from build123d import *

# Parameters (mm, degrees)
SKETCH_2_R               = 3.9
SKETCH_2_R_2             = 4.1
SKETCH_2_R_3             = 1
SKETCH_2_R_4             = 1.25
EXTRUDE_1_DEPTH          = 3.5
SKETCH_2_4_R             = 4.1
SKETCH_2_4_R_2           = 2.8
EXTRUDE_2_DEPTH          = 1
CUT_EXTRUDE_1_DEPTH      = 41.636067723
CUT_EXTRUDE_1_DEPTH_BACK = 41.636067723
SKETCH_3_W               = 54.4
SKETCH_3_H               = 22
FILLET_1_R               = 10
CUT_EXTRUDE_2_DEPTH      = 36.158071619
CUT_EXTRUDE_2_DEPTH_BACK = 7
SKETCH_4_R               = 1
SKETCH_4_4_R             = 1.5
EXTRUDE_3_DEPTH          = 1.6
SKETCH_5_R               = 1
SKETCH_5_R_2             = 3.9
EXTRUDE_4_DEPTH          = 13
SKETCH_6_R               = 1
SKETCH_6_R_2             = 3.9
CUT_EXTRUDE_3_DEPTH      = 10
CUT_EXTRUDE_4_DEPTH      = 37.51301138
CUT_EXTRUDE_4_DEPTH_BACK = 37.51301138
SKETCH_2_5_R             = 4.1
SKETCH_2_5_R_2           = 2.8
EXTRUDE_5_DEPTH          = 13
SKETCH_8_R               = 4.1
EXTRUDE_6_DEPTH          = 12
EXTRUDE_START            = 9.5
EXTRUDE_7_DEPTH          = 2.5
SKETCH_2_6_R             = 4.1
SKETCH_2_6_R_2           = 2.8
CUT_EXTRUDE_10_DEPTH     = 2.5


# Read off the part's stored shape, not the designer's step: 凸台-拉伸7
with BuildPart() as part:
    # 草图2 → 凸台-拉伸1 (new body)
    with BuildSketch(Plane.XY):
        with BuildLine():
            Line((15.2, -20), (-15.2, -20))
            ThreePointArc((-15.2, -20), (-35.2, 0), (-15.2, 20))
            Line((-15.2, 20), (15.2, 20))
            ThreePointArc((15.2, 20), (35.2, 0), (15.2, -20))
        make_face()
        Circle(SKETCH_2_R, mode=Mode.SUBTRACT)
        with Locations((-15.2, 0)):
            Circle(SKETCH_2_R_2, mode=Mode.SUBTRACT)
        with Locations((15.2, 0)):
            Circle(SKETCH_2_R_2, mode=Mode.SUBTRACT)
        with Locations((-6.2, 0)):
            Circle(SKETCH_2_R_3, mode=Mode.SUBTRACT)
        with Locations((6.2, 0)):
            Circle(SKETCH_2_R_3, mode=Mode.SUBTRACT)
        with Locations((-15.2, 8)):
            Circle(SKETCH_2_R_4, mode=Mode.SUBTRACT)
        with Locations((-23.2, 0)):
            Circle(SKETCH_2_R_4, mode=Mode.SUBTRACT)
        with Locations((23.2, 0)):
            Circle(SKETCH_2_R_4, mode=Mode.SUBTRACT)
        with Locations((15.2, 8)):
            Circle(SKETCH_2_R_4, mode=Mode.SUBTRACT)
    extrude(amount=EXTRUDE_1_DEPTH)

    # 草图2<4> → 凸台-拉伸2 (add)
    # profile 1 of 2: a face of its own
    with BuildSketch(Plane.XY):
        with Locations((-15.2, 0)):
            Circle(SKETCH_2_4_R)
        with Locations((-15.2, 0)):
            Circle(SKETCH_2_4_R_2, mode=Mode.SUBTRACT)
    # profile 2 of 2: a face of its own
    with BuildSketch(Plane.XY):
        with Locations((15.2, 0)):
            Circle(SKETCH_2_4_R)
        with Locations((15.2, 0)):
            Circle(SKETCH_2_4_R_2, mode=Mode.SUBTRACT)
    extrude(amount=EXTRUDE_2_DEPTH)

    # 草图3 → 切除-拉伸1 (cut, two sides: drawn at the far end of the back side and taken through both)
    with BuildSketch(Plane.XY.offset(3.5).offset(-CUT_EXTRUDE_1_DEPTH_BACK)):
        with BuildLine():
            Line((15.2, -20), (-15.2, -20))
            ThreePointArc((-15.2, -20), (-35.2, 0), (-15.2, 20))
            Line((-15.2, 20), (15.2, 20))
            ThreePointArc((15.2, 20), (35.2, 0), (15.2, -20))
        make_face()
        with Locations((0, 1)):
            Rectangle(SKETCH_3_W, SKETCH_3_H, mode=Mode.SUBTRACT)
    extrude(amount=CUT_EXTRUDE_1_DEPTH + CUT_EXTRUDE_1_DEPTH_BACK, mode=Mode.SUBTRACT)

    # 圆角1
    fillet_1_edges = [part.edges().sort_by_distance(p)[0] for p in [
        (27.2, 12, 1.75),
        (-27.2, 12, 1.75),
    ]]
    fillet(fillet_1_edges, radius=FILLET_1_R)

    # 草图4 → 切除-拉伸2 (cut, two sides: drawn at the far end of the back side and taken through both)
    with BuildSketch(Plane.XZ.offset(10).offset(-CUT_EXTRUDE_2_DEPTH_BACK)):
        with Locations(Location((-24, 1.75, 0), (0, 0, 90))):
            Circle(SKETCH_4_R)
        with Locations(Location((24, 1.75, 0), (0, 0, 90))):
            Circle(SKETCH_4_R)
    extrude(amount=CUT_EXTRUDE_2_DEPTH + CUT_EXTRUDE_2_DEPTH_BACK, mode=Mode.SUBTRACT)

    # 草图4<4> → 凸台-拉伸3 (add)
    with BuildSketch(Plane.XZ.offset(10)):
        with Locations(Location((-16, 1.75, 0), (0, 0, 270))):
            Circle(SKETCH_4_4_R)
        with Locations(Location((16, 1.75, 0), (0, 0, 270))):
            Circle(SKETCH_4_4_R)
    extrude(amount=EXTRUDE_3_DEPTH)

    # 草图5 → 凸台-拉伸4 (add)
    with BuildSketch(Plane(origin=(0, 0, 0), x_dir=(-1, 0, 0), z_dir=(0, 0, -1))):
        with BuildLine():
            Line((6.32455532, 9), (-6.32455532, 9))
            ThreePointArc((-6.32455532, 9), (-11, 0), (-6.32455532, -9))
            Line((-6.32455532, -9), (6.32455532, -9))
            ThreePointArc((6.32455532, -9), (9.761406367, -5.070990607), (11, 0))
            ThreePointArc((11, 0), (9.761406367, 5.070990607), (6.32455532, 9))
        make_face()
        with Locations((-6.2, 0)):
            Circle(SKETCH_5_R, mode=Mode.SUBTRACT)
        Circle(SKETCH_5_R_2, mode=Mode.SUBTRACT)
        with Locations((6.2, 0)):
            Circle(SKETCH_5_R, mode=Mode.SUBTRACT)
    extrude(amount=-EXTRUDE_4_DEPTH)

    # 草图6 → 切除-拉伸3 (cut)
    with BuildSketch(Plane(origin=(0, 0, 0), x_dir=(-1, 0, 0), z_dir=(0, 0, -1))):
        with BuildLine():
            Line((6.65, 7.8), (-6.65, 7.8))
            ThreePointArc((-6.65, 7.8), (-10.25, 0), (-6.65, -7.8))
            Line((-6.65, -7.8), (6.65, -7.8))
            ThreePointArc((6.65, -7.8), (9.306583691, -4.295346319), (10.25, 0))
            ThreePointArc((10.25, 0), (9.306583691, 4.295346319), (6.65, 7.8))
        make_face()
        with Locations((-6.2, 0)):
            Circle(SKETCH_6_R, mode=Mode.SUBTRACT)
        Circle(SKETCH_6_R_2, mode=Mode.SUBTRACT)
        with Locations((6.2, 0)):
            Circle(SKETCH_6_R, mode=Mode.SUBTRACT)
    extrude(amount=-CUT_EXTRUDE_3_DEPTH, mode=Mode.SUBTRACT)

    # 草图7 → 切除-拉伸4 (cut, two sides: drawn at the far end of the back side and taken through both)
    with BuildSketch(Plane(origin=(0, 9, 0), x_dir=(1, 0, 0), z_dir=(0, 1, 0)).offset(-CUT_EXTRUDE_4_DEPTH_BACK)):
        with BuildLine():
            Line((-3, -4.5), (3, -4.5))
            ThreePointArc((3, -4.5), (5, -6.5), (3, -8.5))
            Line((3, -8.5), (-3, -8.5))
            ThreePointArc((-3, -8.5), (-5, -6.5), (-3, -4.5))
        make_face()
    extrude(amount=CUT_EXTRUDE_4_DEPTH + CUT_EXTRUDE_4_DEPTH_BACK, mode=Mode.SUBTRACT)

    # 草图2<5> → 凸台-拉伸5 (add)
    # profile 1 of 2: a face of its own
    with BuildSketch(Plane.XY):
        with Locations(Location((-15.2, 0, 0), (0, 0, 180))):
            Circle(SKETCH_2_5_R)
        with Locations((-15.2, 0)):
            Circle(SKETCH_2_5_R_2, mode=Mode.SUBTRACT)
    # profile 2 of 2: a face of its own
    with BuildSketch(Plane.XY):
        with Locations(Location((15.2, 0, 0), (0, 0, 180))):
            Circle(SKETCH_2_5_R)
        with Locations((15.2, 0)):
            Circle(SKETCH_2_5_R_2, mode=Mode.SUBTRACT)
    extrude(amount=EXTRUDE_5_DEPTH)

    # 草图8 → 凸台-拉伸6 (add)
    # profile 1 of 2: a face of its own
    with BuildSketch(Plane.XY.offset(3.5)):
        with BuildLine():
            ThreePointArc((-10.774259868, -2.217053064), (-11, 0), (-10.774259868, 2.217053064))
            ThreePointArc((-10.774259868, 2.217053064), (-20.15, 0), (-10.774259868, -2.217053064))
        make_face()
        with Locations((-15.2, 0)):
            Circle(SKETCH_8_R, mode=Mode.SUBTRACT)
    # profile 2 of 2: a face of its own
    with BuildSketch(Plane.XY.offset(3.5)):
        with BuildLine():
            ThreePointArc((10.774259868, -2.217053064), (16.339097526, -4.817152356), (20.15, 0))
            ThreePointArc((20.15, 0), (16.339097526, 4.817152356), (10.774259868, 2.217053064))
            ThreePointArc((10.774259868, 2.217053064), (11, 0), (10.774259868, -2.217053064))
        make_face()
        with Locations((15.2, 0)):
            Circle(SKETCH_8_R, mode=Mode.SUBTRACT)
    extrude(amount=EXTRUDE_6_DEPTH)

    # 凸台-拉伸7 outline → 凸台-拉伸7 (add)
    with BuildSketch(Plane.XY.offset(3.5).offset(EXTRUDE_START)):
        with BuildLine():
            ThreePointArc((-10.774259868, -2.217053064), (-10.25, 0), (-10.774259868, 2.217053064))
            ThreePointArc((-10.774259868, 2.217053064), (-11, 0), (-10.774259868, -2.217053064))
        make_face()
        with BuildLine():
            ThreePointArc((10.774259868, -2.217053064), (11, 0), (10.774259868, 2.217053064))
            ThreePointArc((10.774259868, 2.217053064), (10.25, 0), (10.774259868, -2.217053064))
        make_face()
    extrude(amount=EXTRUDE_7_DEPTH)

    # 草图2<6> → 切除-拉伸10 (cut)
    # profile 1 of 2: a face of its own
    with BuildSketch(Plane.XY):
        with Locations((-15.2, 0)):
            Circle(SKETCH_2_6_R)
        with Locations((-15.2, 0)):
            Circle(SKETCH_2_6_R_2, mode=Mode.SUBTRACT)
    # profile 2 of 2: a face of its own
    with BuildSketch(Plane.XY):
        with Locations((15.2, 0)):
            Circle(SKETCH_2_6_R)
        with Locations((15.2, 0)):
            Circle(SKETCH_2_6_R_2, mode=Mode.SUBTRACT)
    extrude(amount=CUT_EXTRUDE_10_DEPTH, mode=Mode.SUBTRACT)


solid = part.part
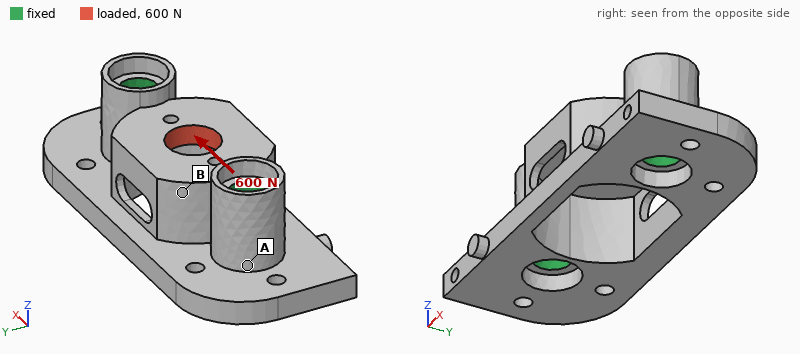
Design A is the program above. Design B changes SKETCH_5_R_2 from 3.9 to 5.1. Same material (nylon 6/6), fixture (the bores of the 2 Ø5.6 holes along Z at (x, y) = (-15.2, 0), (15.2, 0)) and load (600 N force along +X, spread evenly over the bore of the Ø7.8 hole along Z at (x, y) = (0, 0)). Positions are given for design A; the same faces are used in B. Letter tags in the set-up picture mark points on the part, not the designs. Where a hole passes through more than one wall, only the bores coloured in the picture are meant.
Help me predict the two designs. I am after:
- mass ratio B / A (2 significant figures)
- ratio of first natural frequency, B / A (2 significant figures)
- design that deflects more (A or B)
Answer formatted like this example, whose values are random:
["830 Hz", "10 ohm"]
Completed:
["0.98", "1.0", "B"]
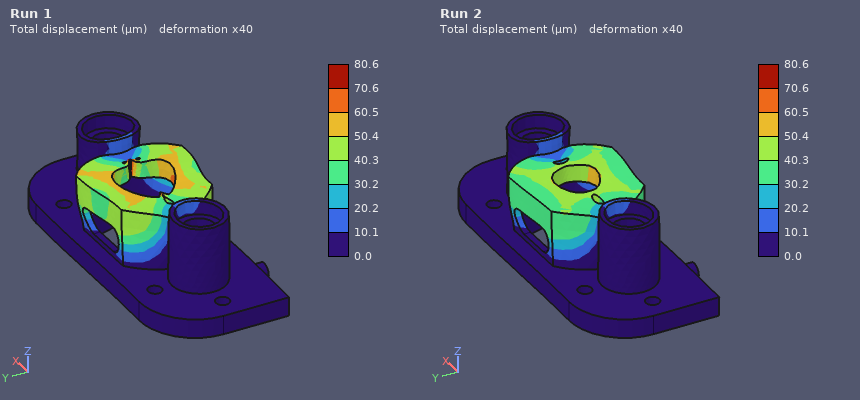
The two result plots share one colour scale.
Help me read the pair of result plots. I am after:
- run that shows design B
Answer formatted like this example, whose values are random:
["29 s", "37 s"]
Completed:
["Run 1"]
